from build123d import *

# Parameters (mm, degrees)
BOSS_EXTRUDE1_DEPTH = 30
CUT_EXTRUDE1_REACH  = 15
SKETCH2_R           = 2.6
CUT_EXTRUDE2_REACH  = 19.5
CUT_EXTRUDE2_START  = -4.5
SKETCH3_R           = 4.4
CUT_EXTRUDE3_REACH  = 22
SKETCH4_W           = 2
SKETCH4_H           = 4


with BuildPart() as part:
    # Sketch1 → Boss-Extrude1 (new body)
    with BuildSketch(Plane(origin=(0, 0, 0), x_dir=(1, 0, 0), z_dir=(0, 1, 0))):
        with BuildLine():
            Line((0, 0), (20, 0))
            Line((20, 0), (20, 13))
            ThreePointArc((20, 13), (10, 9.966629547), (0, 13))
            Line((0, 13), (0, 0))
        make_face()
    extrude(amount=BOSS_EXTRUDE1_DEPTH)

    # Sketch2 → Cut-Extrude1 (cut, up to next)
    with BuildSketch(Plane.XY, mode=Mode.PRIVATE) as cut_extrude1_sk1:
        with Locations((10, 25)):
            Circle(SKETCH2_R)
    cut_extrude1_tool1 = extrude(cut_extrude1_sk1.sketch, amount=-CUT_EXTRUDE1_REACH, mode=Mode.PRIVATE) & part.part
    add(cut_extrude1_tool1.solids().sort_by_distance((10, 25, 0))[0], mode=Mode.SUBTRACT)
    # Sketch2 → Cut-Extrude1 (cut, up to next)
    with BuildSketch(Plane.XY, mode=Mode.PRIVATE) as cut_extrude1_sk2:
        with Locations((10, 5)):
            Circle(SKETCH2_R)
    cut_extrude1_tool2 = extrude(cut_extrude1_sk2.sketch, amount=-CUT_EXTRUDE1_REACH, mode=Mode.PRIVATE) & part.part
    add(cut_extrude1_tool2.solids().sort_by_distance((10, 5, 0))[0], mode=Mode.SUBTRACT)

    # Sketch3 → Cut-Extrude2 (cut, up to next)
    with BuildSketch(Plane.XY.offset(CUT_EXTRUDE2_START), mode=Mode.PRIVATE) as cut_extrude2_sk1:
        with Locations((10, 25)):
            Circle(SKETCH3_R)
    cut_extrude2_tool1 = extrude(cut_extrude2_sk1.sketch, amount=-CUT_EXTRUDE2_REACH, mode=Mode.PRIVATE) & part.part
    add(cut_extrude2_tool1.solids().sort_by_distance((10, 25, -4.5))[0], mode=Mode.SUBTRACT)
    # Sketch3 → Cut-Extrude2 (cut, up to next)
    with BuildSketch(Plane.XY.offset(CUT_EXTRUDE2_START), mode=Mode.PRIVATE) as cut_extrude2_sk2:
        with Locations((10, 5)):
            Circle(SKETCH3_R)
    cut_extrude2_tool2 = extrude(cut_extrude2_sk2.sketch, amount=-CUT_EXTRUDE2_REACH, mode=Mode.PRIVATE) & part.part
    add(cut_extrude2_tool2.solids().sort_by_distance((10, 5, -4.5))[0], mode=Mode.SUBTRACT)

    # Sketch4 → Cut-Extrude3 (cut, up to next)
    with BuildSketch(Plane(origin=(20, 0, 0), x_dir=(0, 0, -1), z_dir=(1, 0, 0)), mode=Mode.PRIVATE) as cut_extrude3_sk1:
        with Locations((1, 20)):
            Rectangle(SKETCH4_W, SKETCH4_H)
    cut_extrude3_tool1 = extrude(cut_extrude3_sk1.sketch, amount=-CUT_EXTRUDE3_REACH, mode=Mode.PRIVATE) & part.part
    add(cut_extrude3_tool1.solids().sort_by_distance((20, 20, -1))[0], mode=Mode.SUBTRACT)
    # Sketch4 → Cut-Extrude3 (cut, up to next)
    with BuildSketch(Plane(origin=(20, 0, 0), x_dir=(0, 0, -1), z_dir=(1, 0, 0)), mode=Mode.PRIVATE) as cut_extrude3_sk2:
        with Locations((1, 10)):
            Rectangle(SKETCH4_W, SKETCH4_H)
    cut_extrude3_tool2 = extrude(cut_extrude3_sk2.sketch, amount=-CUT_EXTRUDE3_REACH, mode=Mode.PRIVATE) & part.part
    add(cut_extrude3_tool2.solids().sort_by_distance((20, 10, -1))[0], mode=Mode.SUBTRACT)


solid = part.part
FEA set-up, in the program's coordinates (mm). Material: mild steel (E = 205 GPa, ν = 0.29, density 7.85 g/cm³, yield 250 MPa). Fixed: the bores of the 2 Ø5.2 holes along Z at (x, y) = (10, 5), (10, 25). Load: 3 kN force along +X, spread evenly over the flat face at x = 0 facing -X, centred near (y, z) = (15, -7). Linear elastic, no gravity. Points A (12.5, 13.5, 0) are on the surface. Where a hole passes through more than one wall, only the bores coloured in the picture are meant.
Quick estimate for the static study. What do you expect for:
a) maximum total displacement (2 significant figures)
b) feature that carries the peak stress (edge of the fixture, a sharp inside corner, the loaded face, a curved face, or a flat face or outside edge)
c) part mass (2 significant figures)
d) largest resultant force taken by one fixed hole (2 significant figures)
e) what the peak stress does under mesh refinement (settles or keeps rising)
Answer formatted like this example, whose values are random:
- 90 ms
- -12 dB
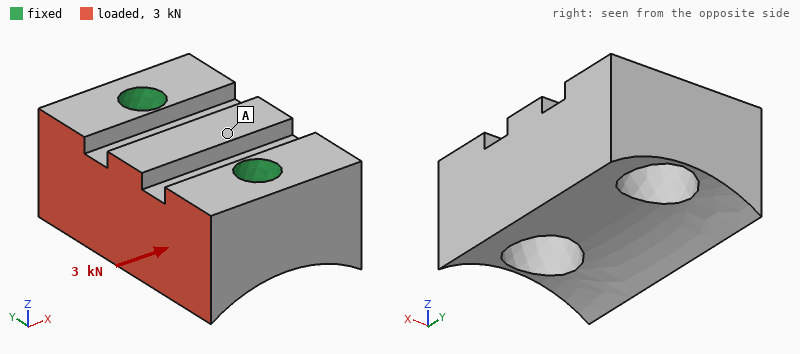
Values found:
- 8.8 µm
- edge of the fixture
- 42 g
- 1.5 kN
- keeps rising
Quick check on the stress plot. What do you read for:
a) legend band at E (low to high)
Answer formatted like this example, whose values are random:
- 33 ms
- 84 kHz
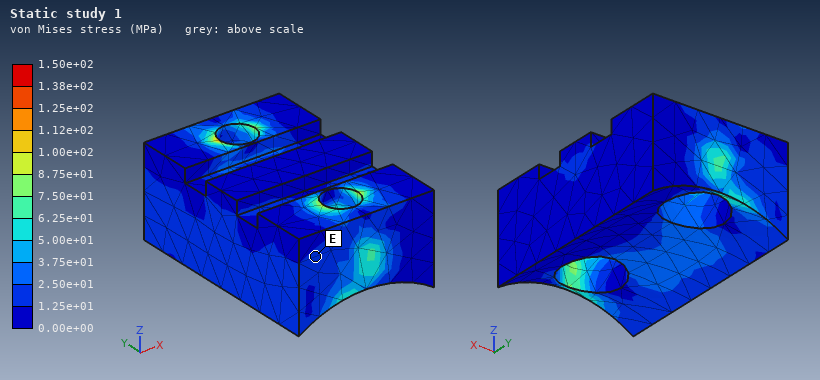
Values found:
- 1.25e+01 to 2.50e+01 MPa
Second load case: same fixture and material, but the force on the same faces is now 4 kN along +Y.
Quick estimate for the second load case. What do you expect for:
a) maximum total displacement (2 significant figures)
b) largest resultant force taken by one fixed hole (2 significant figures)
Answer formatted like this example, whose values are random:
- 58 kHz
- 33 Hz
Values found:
- 6.4 µm
- 2.6 kN
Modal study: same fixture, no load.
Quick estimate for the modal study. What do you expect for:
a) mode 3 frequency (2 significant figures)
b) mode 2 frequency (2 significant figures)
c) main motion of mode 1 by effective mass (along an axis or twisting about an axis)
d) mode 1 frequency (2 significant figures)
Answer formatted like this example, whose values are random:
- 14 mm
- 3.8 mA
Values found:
- 35 kHz
- 35 kHz
- along X
- 19 kHz
